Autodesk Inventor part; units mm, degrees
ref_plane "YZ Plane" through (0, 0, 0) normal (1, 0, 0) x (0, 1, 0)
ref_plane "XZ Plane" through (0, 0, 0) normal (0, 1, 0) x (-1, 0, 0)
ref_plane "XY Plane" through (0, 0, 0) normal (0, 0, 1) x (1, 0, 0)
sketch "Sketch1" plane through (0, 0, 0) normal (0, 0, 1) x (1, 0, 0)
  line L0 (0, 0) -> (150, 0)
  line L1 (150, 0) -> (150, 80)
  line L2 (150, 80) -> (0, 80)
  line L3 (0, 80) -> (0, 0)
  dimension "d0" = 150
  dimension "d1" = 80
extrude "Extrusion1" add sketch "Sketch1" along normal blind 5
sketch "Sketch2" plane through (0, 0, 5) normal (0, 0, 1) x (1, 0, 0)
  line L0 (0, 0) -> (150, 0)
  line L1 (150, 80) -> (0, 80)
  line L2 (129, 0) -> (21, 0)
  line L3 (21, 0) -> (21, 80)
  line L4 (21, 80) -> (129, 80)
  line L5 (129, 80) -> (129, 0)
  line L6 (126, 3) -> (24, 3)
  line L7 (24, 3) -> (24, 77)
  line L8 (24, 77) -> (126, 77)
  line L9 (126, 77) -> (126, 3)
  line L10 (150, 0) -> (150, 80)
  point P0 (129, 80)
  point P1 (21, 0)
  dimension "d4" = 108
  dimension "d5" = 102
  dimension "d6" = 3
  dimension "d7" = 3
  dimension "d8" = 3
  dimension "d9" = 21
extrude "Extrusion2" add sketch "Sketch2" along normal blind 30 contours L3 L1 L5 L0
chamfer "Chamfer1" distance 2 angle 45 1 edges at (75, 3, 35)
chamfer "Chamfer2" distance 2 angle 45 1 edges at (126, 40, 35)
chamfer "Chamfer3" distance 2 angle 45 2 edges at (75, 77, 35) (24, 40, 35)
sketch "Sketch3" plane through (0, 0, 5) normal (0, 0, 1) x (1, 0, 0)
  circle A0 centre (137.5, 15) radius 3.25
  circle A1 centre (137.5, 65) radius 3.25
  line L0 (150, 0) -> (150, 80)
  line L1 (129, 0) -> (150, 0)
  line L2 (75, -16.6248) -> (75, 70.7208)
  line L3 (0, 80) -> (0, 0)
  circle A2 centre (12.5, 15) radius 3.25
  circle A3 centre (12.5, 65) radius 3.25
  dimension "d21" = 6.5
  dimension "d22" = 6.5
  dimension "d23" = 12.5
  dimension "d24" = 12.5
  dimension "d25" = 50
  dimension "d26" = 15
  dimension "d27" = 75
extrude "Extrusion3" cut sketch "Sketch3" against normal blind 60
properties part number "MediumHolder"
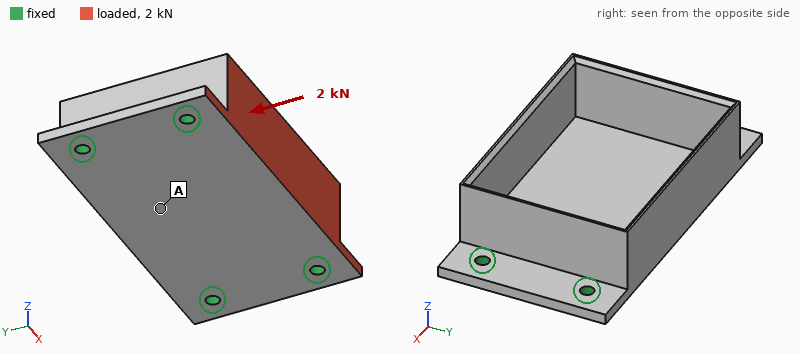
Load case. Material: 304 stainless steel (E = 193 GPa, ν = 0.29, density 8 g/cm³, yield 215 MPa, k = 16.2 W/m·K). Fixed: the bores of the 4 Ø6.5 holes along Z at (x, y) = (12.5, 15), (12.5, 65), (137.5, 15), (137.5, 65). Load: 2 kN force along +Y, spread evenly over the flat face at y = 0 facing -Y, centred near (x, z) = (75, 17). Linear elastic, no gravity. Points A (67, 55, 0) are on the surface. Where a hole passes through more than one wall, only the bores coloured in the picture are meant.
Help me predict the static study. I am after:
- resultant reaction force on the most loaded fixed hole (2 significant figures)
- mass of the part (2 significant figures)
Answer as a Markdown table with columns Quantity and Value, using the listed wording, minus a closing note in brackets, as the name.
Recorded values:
| Quantity | Value |
|---|---|
| resultant reaction force on the most loaded fixed hole | 740 N |
| mass of the part | 730 g |
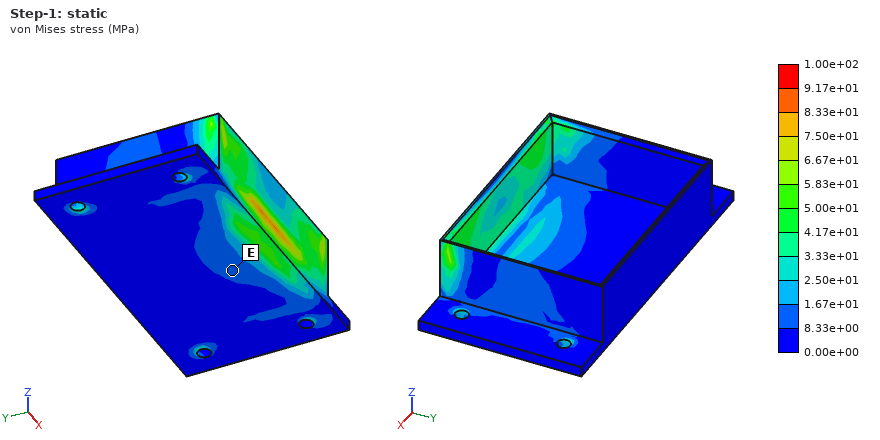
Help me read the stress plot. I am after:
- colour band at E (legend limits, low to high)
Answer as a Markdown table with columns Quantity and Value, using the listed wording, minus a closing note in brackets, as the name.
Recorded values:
| Quantity | Value |
|---|---|
| colour band at E | 8.33e+00 to 1.67e+01 MPa |
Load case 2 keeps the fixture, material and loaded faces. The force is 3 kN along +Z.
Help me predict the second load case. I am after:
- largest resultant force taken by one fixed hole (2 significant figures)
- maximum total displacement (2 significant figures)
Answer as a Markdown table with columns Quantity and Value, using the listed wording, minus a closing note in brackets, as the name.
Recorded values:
| Quantity | Value |
|---|---|
| largest resultant force taken by one fixed hole | 2.2 kN |
| maximum total displacement | 51 µm |
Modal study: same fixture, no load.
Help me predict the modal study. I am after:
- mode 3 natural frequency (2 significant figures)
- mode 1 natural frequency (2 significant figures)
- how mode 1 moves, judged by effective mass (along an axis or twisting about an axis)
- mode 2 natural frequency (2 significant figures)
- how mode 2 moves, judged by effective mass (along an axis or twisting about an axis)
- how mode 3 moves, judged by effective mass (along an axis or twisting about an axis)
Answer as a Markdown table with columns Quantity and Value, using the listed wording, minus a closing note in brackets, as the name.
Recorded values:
| Quantity | Value |
|---|---|
| mode 3 natural frequency | 3200 Hz |
| mode 1 natural frequency | 2600 Hz |
| how mode 1 moves, judged by effective mass | along Z |
| mode 2 natural frequency | 2900 Hz |
| how mode 2 moves, judged by effective mass | along Y |
| how mode 3 moves, judged by effective mass | along Z |
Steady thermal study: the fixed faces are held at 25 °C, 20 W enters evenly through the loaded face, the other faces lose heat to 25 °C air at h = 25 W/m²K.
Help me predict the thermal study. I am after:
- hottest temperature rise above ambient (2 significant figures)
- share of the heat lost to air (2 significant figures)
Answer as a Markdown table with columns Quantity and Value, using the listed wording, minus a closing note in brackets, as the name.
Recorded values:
| Quantity | Value |
|---|---|
| hottest temperature rise above ambient | 66 K |
| share of the heat lost to air | 64 % |
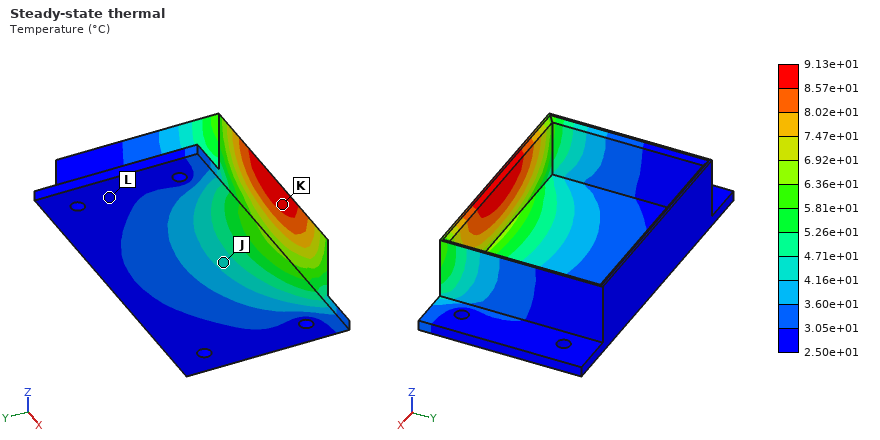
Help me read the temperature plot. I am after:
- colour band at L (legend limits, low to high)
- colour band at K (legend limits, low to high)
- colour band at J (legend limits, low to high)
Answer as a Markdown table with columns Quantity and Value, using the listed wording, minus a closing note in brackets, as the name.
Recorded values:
| Quantity | Value |
|---|---|
| colour band at L | 2.50e+01 to 3.05e+01 °C |
| colour band at K | 8.57e+01 to 9.13e+01 °C |
| colour band at J | 4.16e+01 to 4.71e+01 °C |
